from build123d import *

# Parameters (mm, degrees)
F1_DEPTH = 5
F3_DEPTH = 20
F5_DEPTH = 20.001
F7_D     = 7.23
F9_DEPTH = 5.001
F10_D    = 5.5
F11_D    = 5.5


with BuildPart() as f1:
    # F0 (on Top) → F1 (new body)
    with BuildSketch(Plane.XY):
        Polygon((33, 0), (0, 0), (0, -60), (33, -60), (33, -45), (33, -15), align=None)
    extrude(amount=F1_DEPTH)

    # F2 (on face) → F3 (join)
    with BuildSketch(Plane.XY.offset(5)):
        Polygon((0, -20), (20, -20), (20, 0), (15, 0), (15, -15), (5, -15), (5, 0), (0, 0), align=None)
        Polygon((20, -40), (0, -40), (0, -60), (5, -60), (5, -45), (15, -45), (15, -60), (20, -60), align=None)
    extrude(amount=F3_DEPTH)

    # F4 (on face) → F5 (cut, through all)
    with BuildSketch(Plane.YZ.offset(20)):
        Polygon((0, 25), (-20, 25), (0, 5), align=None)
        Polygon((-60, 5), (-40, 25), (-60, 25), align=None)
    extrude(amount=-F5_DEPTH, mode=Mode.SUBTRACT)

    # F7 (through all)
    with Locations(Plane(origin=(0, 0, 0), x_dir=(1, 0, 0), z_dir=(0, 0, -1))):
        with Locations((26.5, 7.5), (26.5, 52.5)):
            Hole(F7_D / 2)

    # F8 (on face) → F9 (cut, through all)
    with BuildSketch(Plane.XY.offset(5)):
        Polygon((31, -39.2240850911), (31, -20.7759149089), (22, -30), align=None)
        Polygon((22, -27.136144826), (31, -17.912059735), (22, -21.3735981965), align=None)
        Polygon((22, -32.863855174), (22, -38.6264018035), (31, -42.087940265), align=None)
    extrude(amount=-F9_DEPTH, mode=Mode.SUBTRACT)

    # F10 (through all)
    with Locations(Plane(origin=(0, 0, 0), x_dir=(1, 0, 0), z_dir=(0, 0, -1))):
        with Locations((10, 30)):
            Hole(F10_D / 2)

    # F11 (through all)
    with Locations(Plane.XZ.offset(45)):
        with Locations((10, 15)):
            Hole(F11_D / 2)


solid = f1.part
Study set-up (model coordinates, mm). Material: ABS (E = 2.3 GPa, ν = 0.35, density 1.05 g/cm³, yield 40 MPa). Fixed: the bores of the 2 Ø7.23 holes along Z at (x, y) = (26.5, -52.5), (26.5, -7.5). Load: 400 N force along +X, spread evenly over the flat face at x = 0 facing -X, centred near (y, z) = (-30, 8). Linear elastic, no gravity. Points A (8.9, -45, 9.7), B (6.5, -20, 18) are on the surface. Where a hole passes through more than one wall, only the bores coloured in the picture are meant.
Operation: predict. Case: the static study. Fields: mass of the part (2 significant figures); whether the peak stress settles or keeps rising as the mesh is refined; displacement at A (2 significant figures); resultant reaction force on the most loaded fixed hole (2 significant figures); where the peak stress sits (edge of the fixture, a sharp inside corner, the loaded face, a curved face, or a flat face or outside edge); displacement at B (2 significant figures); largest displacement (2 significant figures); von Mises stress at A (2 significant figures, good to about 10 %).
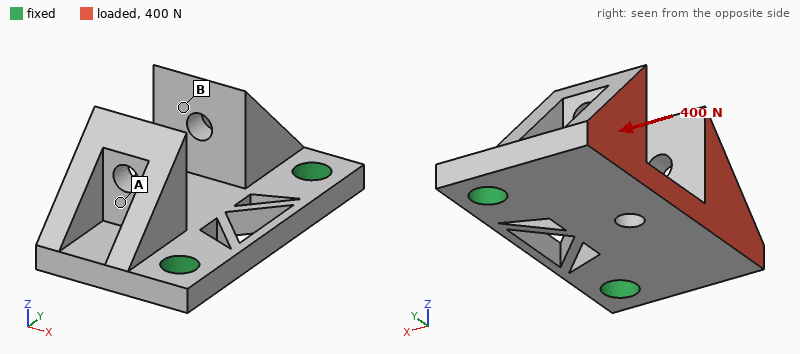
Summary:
15 g
keeps rising
0.25 mm
210 N
edge of the fixture
0.38 mm
0.54 mm
2.9 MPa
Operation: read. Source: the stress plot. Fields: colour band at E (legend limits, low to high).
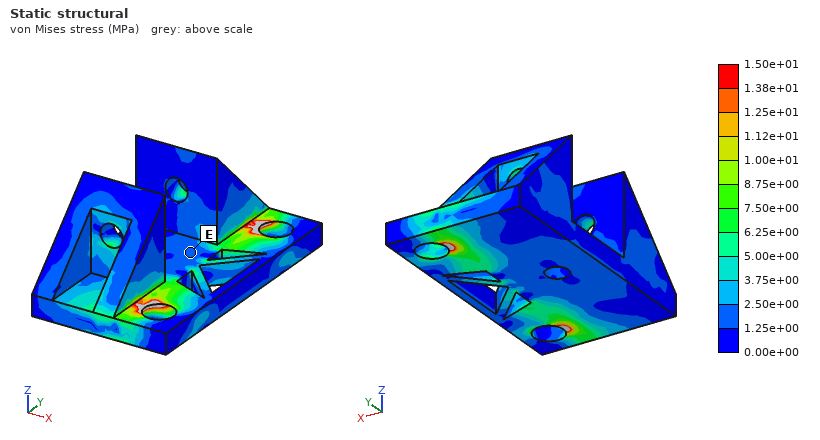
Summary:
1.25e+00 to 2.50e+00 MPa
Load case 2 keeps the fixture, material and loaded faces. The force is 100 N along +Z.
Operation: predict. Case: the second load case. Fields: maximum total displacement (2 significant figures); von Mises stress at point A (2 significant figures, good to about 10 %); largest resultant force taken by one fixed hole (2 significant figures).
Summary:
0.56 mm
1.4 MPa
50 N
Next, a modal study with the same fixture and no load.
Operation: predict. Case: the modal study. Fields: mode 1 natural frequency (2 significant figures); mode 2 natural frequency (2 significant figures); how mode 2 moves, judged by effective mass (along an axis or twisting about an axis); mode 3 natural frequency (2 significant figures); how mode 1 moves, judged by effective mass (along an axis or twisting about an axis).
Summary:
1000 Hz
1800 Hz
twisting about X
2500 Hz
along Z
